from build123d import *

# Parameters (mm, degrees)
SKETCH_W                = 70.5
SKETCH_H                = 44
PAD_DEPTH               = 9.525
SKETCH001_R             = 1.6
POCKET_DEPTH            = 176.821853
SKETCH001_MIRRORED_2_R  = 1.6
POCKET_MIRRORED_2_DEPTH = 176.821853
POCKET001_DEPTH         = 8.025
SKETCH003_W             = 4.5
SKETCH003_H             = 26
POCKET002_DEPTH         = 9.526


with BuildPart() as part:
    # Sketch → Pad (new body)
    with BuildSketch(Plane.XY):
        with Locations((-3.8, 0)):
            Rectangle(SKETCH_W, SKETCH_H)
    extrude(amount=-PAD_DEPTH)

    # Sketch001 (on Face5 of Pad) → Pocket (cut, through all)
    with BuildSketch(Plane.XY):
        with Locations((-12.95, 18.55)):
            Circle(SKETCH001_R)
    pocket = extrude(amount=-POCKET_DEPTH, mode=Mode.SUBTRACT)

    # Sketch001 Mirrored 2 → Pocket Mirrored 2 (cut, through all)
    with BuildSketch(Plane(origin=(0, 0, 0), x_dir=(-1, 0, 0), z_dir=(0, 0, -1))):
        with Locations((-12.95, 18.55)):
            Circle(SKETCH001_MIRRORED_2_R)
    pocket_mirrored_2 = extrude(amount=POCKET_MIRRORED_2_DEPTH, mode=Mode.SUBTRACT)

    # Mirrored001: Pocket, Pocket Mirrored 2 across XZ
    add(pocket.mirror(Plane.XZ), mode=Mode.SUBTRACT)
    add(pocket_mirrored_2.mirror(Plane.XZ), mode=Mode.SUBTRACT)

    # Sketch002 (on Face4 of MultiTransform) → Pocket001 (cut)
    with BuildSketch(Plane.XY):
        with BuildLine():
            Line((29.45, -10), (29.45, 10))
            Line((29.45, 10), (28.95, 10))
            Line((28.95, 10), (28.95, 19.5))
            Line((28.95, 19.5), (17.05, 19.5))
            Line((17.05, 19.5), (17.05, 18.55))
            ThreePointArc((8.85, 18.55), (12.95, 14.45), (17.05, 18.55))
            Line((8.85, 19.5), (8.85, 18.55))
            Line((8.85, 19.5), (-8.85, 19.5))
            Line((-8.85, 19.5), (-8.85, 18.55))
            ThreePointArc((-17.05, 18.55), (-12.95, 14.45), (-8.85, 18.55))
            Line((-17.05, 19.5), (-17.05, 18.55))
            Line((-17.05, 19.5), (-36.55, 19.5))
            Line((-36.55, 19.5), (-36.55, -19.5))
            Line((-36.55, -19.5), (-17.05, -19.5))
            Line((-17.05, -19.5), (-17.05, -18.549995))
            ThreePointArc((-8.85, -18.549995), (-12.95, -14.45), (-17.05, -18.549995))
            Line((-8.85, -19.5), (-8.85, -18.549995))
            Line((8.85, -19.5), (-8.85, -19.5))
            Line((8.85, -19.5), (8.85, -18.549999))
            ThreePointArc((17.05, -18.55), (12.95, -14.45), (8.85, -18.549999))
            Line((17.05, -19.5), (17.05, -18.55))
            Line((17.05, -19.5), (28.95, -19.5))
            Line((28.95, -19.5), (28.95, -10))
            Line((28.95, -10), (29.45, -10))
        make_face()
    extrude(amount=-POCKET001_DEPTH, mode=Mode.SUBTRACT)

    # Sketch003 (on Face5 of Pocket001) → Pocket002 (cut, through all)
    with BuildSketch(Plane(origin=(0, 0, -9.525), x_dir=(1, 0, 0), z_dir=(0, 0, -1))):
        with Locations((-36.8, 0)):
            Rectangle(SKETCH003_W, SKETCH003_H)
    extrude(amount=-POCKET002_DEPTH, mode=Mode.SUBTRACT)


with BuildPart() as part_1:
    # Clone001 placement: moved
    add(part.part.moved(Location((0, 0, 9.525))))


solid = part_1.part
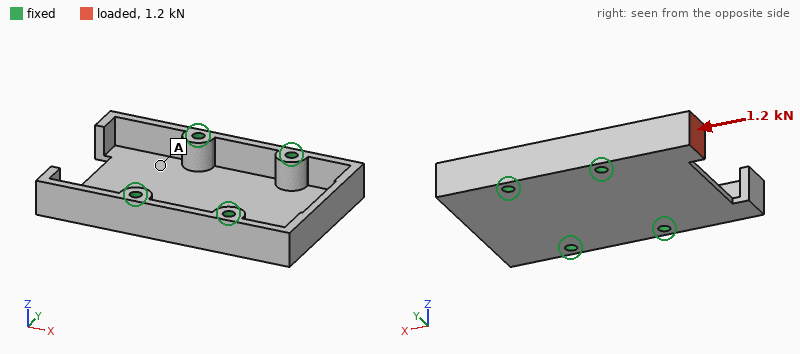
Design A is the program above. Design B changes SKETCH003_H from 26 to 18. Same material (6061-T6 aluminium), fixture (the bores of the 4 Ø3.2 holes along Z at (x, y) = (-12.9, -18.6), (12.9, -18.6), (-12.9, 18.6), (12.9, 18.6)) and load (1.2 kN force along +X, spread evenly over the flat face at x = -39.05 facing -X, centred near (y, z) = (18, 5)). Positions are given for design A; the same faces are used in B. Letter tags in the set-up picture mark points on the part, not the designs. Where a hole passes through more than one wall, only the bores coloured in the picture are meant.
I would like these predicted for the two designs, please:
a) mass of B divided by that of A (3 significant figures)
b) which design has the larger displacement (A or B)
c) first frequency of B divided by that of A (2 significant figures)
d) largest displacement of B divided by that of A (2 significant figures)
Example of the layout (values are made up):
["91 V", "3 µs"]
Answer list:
["1.02", "B", "0.90", "1.4"]
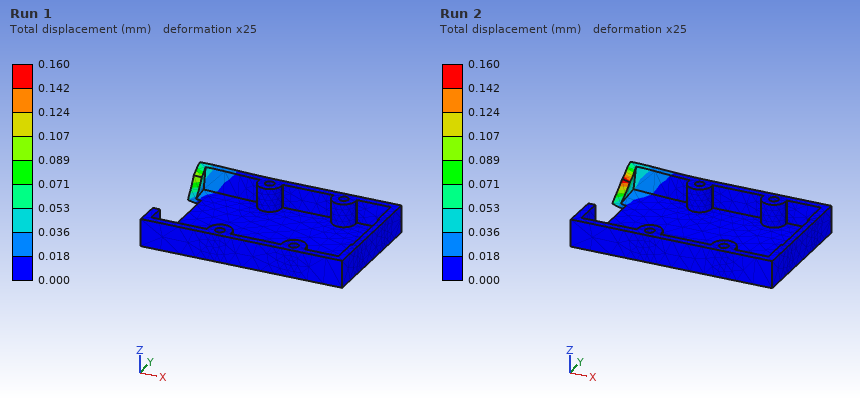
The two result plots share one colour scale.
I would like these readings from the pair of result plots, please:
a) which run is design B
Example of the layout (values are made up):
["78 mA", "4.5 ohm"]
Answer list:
["Run 2"]
